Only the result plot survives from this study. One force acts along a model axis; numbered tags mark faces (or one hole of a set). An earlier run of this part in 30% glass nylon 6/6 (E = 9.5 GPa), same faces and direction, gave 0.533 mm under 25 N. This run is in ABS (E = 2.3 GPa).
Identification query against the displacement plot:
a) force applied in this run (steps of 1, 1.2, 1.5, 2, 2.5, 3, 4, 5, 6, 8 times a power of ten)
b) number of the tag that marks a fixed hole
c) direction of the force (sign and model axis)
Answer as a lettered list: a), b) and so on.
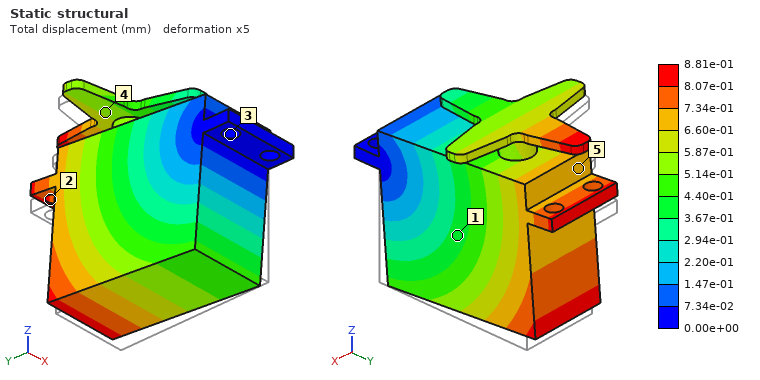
a) 10 N
b) 3
c) +Z
